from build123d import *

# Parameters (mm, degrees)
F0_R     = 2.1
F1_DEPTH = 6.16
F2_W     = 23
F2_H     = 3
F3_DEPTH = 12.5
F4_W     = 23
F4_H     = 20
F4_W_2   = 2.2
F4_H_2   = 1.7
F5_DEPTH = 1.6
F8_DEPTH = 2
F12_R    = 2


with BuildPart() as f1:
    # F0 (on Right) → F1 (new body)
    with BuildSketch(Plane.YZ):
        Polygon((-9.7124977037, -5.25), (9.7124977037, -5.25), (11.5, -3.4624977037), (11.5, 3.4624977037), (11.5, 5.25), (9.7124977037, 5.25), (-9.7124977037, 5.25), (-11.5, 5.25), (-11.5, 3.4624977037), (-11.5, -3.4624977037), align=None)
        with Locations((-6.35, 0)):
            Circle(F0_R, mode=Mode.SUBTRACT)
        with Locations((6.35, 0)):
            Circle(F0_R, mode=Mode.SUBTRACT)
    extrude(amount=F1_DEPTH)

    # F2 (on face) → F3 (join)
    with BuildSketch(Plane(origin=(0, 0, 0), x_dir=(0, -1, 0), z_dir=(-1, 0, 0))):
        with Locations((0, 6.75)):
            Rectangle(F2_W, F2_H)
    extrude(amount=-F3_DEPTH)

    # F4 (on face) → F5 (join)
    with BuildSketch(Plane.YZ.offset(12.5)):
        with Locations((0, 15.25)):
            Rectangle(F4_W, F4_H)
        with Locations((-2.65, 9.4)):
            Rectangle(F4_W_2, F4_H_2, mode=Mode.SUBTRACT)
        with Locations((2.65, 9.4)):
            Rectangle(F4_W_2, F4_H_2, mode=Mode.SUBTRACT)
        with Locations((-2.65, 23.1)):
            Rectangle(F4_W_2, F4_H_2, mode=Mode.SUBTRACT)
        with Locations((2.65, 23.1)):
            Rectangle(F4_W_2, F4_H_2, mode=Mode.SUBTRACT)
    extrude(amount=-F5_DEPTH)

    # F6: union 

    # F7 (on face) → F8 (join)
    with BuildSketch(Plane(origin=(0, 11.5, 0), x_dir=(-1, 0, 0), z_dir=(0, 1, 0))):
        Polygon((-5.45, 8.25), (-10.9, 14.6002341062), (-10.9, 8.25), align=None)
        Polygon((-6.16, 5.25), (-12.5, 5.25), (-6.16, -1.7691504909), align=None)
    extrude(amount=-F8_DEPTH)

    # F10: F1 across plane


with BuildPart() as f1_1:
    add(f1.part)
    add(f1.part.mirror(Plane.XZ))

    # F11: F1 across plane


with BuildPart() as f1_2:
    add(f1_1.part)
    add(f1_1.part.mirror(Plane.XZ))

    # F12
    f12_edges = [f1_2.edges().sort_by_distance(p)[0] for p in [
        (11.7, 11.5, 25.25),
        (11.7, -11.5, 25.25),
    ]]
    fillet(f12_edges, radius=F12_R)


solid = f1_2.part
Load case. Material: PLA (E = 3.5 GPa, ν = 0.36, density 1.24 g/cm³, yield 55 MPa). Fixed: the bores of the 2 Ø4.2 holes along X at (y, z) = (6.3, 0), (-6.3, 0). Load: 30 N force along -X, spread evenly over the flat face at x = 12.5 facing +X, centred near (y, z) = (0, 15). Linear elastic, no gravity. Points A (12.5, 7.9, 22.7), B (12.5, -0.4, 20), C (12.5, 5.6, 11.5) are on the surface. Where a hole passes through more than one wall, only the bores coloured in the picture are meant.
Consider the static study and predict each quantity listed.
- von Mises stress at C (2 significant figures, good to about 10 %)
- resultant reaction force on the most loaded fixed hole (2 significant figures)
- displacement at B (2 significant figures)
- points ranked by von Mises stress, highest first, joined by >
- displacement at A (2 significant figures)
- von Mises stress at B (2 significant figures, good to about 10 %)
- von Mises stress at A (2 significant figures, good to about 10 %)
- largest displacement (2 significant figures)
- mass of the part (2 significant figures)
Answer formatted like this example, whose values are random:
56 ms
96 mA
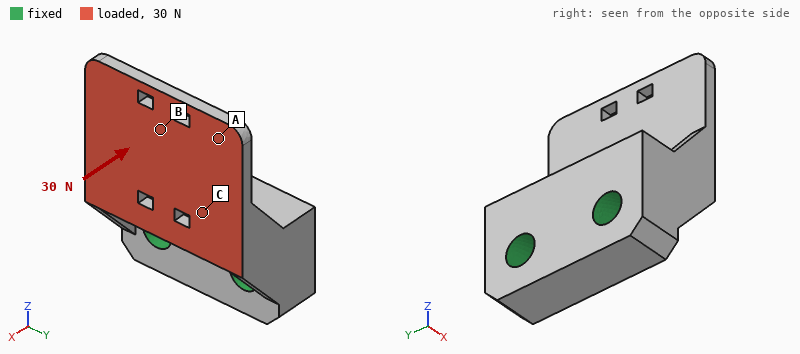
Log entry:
7.9 MPa
16 N
0.27 mm
C > B > A
0.31 mm
4.4 MPa
1.8 MPa
0.43 mm
3.6 g
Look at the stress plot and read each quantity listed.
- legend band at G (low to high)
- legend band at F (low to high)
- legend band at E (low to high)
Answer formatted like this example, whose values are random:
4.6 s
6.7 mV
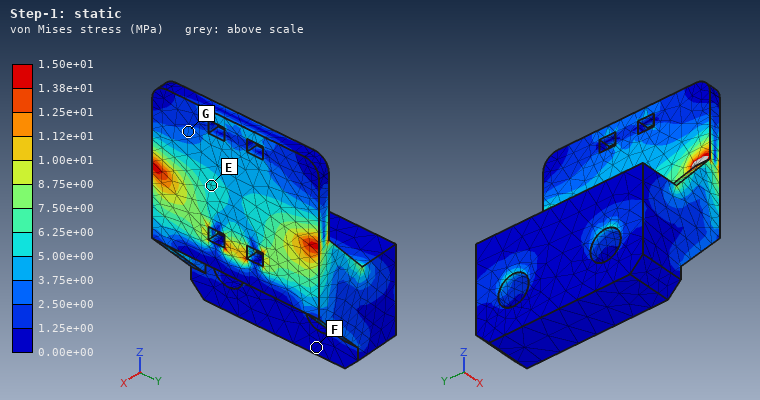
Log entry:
2.50e+00 to 3.75e+00 MPa
0.00e+00 to 1.25e+00 MPa
5.00e+00 to 6.25e+00 MPa
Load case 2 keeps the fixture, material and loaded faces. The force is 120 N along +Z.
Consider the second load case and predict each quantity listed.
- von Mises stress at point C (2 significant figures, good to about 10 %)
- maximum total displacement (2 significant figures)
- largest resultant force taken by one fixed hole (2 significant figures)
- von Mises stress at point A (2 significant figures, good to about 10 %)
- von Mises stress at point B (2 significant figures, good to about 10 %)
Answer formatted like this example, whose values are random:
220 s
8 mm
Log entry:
6.5 MPa
0.40 mm
61 N
2.1 MPa
3.3 MPa
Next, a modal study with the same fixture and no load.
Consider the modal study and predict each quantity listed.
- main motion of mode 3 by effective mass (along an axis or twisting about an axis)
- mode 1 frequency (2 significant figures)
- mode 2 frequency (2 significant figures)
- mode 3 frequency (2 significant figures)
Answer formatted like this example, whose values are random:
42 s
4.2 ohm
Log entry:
along Y
1800 Hz
3600 Hz
6400 Hz
